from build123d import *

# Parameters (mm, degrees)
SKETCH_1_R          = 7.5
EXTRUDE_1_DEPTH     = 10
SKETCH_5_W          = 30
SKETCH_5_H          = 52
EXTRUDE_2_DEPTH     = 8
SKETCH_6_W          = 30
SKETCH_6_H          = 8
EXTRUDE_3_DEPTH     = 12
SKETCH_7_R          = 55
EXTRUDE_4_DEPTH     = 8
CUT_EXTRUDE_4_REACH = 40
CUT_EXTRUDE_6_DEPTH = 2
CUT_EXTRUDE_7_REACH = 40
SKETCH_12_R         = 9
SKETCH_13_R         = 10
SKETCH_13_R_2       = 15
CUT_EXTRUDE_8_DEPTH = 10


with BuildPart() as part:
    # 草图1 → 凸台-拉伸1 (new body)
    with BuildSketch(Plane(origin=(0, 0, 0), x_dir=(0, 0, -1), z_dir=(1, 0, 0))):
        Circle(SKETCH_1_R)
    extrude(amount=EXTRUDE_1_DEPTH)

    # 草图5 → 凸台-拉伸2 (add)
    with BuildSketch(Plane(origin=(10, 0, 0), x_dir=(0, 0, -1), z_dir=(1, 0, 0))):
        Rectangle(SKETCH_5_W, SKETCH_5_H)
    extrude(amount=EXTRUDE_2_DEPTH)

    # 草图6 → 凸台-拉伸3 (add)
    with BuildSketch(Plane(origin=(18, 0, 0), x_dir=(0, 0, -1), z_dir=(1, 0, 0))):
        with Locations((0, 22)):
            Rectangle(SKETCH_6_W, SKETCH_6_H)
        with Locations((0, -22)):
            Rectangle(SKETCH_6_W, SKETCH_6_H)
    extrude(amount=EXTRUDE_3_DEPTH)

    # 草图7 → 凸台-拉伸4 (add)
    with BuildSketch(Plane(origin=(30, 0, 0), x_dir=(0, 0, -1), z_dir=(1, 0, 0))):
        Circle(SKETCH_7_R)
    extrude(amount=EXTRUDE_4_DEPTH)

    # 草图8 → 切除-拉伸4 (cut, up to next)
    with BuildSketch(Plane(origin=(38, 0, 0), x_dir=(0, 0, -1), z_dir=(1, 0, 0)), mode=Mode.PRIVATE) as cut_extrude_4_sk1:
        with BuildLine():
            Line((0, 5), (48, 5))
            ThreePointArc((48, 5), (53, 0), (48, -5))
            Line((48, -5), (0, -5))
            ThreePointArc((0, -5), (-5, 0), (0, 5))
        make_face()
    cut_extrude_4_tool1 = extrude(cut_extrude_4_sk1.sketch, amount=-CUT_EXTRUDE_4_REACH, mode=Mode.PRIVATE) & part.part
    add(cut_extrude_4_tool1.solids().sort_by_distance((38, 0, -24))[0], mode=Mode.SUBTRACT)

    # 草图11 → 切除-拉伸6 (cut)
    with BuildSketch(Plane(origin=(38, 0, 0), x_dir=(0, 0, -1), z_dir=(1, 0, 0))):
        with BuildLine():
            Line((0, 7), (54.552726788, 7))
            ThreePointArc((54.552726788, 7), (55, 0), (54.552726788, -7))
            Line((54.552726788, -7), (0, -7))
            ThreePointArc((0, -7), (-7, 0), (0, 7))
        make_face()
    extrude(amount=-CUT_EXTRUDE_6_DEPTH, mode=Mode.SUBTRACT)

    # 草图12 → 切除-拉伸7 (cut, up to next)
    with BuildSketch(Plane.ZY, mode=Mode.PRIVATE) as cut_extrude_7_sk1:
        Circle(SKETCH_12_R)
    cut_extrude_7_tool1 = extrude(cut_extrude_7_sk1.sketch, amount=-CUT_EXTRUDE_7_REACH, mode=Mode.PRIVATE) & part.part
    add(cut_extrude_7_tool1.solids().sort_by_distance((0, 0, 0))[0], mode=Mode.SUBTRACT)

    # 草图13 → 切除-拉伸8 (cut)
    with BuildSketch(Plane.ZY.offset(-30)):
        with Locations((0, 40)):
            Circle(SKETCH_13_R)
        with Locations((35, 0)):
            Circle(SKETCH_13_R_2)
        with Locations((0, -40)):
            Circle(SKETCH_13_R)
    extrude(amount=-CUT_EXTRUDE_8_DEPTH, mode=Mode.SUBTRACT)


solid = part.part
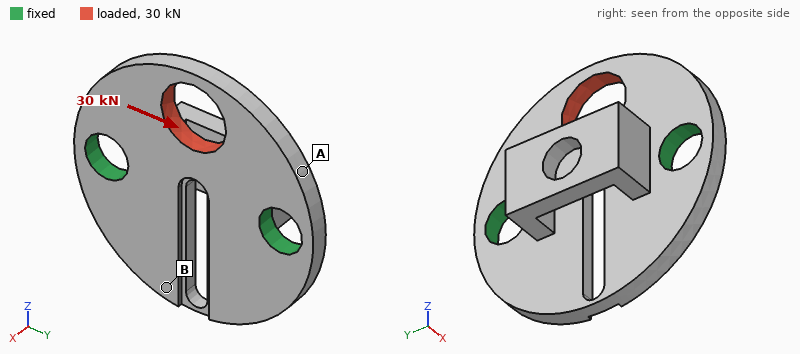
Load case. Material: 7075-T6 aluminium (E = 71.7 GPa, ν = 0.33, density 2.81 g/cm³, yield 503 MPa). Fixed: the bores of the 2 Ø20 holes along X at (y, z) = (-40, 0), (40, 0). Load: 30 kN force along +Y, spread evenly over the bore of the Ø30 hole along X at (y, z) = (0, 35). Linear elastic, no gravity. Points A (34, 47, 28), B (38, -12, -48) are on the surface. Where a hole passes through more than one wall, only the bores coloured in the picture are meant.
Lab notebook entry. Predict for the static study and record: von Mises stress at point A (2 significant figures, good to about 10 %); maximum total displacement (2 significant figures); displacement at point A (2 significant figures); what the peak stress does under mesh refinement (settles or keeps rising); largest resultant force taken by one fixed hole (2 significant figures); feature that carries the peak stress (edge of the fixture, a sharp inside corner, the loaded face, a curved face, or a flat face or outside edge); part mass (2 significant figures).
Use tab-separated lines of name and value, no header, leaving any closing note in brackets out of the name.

von Mises stress at point A	67 MPa
maximum total displacement	0.14 mm
displacement at point A	0.048 mm
what the peak stress does under mesh refinement	keeps rising
largest resultant force taken by one fixed hole	17 kN
feature that carries the peak stress	a sharp inside corner
part mass	210 g
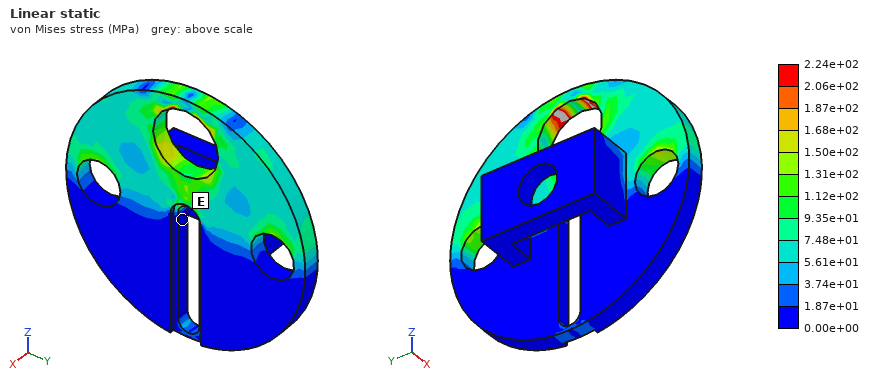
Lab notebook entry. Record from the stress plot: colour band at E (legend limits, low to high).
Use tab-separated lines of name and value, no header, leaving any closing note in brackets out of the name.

colour band at E	0.00e+00 to 1.87e+01 MPa
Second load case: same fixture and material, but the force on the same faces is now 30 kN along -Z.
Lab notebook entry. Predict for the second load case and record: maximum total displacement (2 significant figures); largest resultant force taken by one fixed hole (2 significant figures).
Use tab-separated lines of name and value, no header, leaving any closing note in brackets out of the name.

maximum total displacement	0.11 mm
largest resultant force taken by one fixed hole	16 kN
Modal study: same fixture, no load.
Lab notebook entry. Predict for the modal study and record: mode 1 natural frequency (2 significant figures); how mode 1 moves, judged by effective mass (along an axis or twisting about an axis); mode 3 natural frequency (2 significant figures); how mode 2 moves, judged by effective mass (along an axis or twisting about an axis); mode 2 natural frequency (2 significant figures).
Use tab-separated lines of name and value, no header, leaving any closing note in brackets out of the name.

mode 1 natural frequency	3300 Hz
how mode 1 moves, judged by effective mass	twisting about Y
mode 3 natural frequency	6100 Hz
how mode 2 moves, judged by effective mass	along X
mode 2 natural frequency	3900 Hz
